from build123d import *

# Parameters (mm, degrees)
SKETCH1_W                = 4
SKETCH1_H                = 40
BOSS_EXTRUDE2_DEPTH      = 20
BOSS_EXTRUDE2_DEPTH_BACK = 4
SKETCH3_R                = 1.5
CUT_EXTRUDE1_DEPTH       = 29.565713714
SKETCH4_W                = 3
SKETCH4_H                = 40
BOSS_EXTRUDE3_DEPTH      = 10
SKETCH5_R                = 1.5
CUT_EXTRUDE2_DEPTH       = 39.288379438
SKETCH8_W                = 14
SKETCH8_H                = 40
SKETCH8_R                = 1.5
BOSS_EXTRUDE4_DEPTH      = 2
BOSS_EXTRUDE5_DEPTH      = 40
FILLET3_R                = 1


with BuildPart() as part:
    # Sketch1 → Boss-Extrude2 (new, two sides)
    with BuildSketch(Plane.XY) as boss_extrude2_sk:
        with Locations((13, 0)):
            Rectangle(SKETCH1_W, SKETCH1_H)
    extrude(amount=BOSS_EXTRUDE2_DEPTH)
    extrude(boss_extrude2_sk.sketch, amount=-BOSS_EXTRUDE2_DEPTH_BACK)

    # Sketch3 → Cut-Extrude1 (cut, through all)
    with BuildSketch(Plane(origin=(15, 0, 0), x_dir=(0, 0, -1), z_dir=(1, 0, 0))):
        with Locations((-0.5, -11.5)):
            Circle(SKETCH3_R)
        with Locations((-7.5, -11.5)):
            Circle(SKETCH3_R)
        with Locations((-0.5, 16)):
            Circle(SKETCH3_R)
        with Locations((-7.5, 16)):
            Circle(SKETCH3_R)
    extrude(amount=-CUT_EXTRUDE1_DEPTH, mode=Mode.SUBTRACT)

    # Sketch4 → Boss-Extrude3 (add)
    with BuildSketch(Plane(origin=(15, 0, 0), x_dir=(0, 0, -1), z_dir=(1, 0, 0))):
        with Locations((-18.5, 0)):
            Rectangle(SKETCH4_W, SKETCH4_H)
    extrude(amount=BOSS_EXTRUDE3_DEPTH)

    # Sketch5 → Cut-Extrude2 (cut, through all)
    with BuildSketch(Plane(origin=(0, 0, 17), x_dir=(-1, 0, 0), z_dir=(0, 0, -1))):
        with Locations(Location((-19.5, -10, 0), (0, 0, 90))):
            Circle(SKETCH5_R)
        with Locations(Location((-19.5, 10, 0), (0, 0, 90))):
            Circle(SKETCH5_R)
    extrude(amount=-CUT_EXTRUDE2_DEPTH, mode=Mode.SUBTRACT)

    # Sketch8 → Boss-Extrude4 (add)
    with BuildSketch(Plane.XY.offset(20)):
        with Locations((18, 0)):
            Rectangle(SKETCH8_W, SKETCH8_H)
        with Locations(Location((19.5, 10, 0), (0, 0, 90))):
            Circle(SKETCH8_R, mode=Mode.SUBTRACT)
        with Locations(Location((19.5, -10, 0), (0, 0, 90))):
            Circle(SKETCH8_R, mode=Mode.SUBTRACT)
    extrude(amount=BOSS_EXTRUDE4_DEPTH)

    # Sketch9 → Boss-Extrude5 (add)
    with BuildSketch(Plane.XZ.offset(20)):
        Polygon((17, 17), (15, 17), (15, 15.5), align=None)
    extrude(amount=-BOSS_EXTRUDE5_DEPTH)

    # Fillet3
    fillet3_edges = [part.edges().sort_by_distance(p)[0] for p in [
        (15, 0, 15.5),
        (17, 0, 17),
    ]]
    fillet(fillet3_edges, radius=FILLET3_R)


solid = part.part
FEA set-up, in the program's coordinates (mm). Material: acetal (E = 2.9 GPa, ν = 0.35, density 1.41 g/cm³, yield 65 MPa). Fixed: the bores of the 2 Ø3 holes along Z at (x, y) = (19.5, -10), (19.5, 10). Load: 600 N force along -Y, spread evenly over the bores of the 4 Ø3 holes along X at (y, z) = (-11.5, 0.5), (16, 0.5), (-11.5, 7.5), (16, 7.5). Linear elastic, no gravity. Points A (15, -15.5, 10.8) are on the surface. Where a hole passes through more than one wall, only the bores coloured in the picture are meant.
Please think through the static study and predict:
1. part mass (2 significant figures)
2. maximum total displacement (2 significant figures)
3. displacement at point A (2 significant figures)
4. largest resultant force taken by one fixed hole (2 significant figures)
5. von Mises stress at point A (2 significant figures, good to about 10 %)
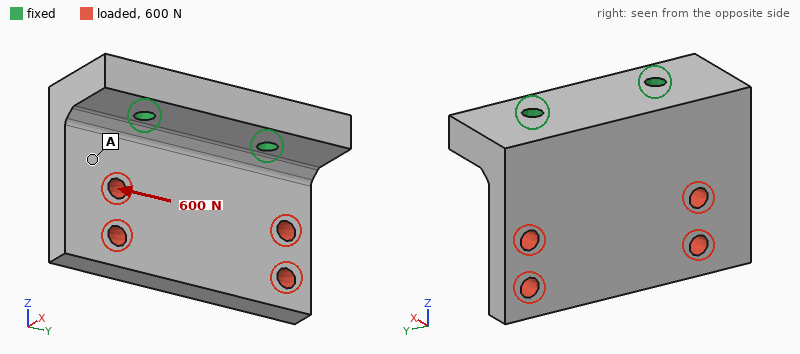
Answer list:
8.5 g
0.42 mm
0.20 mm
510 N
10 MPa
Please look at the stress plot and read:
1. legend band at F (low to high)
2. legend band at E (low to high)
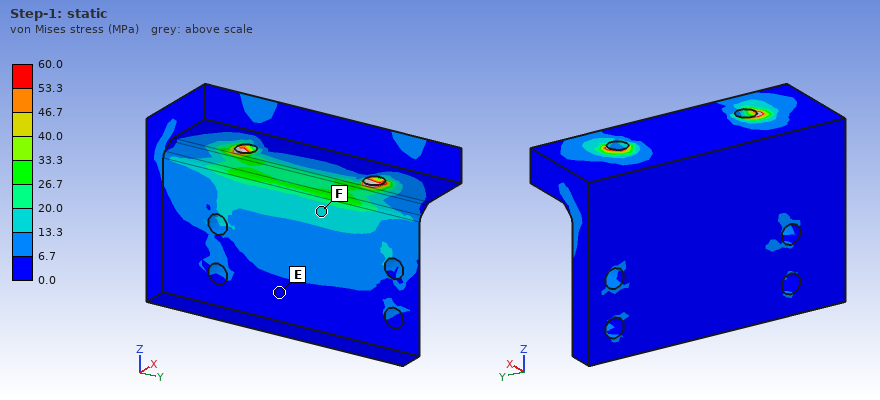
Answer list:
13.3 to 20.0 MPa
0.0 to 6.7 MPa
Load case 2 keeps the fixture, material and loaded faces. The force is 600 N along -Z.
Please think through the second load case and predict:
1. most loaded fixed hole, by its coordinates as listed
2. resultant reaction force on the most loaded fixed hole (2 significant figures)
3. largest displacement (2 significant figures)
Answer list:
(19.5, 10)
360 N
0.46 mm
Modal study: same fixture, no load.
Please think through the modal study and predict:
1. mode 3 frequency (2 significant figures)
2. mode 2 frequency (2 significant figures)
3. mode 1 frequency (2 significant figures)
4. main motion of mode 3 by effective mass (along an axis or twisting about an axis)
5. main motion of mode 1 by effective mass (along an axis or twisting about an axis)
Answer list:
3900 Hz
2500 Hz
1500 Hz
along Y
along X
